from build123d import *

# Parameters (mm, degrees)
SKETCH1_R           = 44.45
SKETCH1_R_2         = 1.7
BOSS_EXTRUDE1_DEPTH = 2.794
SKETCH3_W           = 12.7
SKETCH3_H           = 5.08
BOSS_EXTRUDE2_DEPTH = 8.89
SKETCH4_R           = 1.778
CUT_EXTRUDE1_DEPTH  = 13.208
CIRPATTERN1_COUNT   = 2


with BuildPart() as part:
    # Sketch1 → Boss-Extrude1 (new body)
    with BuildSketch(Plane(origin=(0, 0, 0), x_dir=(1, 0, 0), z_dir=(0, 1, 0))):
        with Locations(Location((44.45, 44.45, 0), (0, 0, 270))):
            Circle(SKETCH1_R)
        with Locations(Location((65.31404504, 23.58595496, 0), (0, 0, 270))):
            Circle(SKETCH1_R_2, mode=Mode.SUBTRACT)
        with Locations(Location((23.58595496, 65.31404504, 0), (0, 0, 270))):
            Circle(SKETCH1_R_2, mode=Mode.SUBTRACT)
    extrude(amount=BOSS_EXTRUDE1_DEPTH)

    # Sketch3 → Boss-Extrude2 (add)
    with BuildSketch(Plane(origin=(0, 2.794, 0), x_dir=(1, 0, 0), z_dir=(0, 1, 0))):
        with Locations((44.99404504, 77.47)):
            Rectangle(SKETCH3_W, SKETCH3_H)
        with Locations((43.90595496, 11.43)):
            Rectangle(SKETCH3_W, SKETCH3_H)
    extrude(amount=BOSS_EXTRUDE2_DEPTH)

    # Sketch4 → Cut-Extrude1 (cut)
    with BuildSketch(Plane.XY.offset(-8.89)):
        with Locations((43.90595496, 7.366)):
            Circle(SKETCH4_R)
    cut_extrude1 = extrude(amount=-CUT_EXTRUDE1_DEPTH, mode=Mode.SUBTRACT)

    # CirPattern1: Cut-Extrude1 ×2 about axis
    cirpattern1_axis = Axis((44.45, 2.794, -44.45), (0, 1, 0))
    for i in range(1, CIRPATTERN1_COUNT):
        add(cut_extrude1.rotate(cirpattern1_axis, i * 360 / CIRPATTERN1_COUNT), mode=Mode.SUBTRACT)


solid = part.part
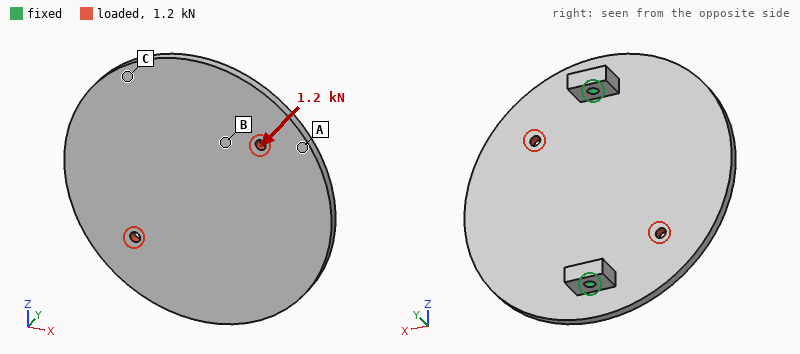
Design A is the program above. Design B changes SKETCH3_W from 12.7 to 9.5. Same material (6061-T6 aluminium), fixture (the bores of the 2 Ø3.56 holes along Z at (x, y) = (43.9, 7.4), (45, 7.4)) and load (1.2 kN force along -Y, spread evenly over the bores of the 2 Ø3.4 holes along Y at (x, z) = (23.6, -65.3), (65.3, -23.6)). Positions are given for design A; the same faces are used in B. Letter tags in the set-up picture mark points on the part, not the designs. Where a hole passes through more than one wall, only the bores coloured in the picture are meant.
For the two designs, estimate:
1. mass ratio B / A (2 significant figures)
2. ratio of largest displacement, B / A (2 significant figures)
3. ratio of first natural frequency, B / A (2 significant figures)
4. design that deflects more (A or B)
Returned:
0.98
1.1
0.91
B
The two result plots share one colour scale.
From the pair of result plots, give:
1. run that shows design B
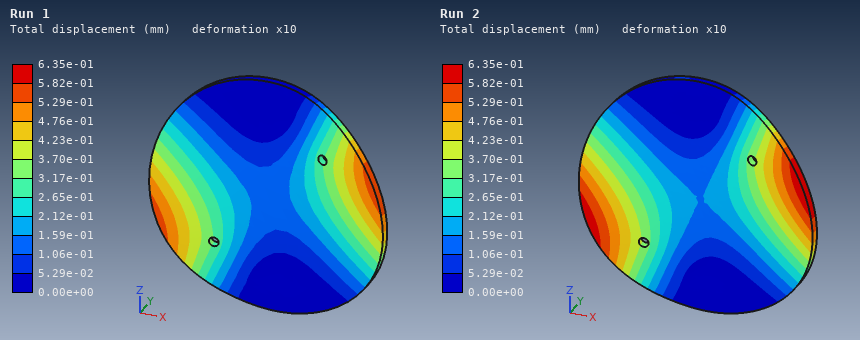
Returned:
Run 2
